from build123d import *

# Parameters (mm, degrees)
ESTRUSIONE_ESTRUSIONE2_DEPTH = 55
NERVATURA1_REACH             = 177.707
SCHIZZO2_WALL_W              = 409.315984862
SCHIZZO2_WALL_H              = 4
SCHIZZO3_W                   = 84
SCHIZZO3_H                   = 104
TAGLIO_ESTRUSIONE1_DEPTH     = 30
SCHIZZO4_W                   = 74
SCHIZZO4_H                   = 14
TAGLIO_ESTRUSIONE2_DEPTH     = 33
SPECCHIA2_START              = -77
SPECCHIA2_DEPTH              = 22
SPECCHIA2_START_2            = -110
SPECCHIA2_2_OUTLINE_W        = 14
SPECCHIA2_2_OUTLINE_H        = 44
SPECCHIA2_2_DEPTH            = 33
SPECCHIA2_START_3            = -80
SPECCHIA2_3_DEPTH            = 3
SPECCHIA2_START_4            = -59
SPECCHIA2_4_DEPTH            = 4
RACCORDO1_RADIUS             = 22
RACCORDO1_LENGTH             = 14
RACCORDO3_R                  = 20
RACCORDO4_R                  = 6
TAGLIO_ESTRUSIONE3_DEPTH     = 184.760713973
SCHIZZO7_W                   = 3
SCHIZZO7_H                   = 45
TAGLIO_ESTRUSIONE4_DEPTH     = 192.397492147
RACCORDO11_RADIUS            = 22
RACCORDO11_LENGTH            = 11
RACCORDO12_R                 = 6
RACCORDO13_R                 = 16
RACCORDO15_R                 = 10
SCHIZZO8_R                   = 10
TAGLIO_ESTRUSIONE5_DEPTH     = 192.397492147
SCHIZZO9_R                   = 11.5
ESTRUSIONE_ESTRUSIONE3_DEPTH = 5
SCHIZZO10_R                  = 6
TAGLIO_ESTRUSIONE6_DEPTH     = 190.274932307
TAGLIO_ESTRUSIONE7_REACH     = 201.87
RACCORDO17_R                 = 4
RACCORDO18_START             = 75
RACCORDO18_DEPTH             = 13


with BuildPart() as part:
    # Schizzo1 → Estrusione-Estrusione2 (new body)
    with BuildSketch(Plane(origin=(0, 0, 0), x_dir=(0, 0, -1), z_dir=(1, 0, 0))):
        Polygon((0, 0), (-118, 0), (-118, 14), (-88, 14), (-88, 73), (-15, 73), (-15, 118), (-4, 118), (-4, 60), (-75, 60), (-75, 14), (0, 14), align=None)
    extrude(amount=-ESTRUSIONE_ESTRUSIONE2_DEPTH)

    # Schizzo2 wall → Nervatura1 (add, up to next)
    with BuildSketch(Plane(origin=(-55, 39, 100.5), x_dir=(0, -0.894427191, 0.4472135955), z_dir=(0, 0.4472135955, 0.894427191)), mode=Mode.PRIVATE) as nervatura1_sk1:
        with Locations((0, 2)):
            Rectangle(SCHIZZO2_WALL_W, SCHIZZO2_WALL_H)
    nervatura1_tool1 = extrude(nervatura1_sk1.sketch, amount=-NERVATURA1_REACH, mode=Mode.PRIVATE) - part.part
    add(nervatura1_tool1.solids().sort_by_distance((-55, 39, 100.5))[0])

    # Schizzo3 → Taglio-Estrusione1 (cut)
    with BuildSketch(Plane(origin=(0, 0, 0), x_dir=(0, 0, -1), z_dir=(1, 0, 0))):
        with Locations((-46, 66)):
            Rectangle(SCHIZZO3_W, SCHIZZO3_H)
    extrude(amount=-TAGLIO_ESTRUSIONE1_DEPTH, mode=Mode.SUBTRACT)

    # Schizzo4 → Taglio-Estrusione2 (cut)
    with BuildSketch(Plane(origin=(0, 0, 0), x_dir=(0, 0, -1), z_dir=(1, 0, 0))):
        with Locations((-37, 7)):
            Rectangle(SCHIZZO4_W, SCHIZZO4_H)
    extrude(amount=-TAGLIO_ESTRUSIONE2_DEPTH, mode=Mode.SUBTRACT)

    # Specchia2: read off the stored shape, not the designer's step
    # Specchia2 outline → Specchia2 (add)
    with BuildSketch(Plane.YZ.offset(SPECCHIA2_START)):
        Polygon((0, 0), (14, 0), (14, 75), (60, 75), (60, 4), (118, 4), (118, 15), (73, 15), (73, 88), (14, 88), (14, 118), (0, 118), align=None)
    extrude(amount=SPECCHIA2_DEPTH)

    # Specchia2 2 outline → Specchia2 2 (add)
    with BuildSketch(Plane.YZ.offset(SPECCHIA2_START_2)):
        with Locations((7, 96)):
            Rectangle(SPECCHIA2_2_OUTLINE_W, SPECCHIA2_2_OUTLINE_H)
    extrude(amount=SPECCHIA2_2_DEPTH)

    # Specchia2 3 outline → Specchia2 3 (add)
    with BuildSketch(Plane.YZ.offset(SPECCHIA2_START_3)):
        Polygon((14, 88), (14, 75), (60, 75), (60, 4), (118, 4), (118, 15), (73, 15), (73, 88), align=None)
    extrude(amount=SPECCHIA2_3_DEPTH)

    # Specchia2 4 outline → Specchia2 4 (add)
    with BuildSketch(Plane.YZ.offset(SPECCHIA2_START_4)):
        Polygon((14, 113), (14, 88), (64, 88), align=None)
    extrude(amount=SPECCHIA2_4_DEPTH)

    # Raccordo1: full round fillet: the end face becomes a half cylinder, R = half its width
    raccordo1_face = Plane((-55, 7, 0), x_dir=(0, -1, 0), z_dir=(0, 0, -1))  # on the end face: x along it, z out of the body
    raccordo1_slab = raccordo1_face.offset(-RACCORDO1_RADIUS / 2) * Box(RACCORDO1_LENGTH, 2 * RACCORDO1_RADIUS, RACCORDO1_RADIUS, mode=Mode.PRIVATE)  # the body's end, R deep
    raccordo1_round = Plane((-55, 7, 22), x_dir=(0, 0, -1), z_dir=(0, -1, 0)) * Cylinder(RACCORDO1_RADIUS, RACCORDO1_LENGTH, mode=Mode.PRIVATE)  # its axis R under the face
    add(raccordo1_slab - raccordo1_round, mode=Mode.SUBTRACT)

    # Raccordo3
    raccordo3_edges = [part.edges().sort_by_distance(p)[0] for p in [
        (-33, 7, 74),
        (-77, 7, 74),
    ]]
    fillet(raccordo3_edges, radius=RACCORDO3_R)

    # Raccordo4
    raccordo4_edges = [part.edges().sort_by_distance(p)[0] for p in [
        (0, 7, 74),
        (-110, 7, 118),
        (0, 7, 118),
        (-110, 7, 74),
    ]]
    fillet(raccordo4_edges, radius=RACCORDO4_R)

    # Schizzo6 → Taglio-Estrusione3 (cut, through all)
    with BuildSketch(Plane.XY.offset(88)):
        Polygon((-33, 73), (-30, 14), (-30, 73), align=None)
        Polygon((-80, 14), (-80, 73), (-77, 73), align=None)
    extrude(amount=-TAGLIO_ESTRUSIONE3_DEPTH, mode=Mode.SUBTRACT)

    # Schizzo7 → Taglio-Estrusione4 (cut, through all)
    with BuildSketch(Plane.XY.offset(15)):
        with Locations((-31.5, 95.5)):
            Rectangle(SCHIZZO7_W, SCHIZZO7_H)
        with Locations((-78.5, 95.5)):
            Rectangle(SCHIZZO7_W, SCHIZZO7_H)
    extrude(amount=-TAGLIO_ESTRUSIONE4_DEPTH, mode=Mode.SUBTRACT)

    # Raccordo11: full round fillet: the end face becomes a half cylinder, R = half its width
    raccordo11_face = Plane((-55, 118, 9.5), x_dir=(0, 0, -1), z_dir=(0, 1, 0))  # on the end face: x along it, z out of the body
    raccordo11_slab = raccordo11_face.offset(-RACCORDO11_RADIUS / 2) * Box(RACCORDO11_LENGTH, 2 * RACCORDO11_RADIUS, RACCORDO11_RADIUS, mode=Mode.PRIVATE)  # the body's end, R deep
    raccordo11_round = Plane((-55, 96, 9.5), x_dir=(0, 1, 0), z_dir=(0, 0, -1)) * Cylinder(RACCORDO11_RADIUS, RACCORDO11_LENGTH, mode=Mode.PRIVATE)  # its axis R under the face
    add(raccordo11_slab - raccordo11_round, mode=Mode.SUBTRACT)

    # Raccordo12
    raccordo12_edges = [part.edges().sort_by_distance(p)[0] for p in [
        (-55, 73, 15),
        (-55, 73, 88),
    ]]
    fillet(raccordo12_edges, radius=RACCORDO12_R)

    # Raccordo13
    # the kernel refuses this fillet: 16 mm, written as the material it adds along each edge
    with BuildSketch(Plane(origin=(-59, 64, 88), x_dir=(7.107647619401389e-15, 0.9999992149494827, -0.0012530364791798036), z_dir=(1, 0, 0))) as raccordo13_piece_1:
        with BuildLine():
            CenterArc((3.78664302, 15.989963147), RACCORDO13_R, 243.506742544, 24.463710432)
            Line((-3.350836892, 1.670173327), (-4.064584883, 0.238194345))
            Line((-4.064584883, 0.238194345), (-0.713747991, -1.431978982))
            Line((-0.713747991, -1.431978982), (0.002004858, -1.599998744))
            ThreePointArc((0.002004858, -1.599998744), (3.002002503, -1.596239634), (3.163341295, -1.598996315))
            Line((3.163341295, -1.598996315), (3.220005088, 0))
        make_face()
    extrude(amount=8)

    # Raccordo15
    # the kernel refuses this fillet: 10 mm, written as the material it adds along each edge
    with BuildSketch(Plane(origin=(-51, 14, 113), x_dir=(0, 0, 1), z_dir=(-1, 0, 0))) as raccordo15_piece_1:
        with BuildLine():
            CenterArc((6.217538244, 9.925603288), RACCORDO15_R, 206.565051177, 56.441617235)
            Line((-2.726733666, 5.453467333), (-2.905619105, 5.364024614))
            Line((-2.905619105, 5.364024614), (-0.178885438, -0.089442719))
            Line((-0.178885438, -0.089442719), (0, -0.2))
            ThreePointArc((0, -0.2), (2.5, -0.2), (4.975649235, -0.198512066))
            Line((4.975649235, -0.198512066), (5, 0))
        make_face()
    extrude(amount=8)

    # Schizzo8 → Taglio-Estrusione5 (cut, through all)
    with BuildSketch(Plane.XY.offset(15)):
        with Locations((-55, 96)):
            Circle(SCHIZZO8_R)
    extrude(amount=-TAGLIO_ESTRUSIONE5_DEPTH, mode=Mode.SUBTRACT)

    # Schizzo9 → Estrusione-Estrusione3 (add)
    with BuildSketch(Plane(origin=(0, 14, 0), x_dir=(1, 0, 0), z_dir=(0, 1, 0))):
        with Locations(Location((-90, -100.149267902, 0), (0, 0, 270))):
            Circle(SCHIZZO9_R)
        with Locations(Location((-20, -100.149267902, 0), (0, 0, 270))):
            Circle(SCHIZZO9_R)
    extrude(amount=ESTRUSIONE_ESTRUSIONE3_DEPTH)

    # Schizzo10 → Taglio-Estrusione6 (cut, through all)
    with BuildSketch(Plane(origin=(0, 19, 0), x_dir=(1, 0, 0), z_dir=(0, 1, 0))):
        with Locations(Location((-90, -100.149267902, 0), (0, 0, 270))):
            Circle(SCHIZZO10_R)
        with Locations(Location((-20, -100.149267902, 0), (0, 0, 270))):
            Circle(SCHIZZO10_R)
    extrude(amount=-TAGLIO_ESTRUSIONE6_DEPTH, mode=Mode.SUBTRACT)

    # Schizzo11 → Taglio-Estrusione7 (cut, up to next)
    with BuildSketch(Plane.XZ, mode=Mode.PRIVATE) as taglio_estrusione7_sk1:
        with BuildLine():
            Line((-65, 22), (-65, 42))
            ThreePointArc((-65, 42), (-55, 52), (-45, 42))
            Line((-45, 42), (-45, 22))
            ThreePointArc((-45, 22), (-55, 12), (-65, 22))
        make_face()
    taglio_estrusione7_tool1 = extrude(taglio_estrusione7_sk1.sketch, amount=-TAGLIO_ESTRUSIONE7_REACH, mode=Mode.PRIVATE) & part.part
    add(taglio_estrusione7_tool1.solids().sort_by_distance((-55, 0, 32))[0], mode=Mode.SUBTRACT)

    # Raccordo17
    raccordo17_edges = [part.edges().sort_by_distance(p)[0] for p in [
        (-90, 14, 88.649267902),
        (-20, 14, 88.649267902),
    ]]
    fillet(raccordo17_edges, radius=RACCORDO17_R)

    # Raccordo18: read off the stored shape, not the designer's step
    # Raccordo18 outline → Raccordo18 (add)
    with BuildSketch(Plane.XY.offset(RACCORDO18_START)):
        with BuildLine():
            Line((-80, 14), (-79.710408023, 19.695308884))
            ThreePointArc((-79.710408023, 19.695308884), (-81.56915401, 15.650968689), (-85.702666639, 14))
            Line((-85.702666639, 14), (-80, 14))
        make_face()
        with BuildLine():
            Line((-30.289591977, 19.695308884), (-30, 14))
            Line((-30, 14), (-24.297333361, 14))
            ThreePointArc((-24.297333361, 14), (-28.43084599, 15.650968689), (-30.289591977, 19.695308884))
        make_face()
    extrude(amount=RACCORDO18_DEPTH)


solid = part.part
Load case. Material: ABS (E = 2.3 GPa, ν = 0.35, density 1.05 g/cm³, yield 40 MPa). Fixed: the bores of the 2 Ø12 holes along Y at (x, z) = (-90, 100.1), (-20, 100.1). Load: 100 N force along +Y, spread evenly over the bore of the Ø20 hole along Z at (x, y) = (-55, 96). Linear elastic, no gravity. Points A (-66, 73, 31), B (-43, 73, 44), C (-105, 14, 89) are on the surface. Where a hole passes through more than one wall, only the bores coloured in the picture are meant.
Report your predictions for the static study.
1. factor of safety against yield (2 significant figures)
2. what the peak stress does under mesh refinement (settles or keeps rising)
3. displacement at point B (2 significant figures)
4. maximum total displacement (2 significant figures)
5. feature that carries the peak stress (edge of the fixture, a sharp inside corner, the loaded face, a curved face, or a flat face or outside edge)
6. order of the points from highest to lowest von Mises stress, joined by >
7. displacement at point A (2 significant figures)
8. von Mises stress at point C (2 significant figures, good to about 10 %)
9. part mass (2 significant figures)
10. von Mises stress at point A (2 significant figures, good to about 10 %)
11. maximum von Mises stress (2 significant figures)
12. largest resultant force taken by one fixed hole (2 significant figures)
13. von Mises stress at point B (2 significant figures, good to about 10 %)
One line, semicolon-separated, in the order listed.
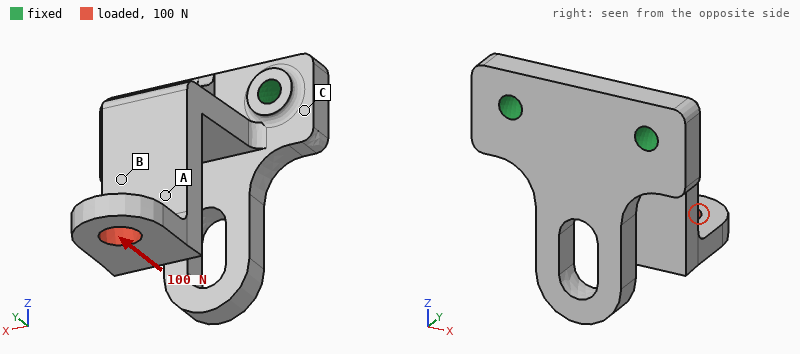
5.2; settles; 0.80 mm; 2.2 mm; a curved face; B > A > C; 1.1 mm; 0.60 MPa; 210 g; 1.7 MPa; 7.6 MPa; 56 N; 2.7 MPa
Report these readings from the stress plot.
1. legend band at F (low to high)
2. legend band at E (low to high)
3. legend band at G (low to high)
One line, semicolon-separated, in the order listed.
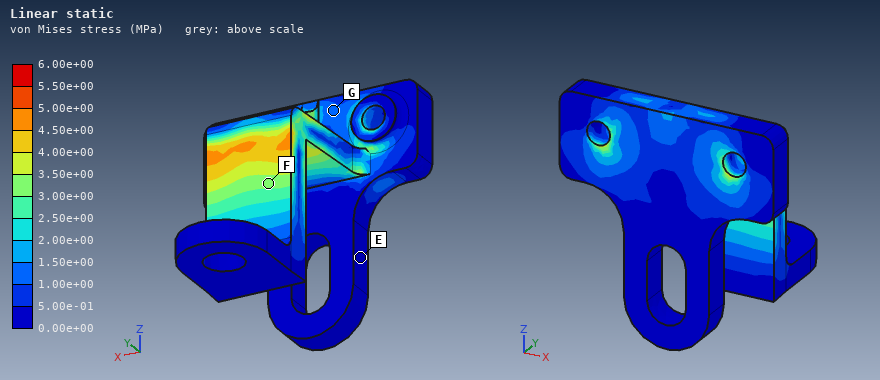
3.00e+00 to 3.50e+00 MPa; 0.00e+00 to 5.00e-01 MPa; 1.00e+00 to 1.50e+00 MPa
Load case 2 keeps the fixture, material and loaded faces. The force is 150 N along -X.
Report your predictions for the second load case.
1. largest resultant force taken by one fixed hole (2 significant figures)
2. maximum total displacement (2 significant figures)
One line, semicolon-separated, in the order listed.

300 N; 1.9 mm
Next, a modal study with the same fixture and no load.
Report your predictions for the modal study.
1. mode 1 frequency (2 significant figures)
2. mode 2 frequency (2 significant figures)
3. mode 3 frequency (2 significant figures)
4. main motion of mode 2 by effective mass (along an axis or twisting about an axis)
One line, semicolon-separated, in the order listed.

190 Hz; 280 Hz; 500 Hz; along X
